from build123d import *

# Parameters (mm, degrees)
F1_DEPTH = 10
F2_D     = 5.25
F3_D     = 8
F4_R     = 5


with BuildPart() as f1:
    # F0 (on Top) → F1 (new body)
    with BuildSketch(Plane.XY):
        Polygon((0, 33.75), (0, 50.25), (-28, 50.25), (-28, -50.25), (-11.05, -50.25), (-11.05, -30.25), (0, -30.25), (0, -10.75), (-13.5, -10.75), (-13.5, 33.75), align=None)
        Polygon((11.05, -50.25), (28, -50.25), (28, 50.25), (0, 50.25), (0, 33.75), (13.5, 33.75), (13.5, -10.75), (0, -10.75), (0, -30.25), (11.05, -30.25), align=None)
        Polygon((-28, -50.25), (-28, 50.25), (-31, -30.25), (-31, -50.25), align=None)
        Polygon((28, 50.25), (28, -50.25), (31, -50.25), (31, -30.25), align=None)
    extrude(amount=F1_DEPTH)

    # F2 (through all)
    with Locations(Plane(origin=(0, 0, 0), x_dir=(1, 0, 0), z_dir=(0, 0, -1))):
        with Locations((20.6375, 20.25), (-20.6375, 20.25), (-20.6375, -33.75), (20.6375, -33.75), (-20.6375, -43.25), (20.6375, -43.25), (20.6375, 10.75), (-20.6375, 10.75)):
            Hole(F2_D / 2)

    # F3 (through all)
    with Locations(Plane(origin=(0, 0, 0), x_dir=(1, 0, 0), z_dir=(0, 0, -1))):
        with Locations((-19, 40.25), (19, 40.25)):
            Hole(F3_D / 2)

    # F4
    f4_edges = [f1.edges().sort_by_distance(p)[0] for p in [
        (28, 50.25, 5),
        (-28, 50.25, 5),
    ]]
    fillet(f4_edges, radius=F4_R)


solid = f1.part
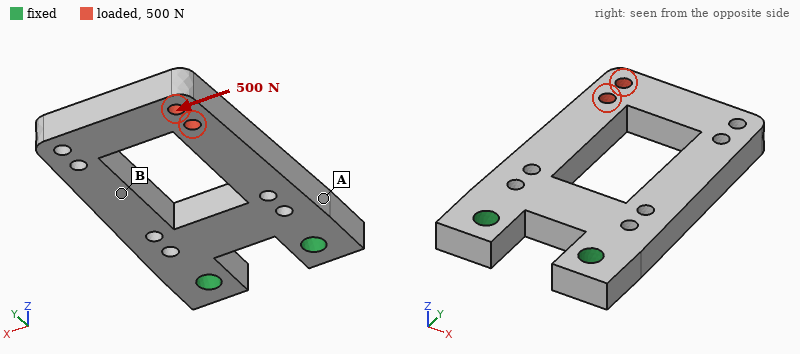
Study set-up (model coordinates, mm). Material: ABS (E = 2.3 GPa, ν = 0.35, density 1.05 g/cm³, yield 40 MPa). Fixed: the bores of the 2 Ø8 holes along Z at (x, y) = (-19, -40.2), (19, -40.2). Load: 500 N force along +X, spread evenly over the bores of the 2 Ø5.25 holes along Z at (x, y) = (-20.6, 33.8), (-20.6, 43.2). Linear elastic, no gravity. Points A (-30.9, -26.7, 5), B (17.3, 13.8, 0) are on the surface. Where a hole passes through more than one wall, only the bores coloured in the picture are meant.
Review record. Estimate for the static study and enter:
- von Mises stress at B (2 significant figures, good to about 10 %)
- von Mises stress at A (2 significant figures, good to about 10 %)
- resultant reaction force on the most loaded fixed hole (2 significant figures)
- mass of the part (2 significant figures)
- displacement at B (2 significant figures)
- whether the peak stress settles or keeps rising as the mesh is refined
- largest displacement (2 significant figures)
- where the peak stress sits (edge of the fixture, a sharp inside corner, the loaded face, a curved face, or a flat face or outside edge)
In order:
3.3 MPa
7.0 MPa
790 N
43 g
0.59 mm
keeps rising
1.1 mm
a sharp inside corner
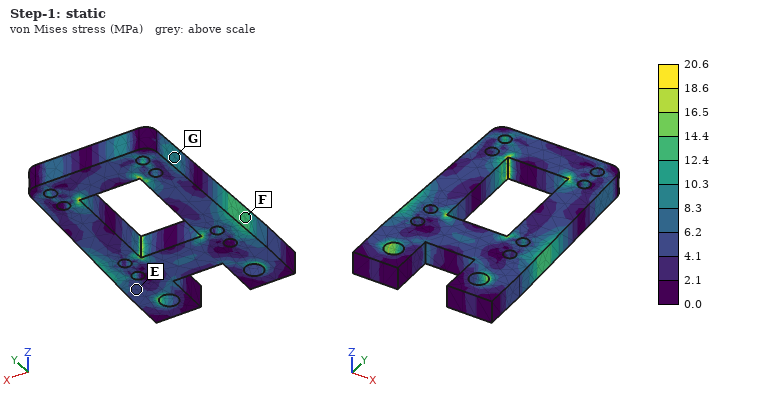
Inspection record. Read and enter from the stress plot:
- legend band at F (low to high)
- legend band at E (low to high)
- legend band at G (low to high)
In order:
12.4 to 14.4 MPa
4.1 to 6.2 MPa
8.3 to 10.3 MPa
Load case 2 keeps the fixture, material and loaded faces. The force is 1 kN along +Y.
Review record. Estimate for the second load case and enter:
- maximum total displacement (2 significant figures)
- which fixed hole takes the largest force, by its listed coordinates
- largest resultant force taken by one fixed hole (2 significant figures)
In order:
0.30 mm
(-19, -40.2)
980 N
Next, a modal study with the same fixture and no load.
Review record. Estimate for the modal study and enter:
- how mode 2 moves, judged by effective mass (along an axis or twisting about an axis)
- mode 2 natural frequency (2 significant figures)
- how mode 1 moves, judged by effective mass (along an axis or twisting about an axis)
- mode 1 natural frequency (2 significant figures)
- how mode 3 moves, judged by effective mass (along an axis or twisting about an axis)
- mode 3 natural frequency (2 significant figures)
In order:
twisting about Y
770 Hz
along Z
280 Hz
along X
900 Hz
